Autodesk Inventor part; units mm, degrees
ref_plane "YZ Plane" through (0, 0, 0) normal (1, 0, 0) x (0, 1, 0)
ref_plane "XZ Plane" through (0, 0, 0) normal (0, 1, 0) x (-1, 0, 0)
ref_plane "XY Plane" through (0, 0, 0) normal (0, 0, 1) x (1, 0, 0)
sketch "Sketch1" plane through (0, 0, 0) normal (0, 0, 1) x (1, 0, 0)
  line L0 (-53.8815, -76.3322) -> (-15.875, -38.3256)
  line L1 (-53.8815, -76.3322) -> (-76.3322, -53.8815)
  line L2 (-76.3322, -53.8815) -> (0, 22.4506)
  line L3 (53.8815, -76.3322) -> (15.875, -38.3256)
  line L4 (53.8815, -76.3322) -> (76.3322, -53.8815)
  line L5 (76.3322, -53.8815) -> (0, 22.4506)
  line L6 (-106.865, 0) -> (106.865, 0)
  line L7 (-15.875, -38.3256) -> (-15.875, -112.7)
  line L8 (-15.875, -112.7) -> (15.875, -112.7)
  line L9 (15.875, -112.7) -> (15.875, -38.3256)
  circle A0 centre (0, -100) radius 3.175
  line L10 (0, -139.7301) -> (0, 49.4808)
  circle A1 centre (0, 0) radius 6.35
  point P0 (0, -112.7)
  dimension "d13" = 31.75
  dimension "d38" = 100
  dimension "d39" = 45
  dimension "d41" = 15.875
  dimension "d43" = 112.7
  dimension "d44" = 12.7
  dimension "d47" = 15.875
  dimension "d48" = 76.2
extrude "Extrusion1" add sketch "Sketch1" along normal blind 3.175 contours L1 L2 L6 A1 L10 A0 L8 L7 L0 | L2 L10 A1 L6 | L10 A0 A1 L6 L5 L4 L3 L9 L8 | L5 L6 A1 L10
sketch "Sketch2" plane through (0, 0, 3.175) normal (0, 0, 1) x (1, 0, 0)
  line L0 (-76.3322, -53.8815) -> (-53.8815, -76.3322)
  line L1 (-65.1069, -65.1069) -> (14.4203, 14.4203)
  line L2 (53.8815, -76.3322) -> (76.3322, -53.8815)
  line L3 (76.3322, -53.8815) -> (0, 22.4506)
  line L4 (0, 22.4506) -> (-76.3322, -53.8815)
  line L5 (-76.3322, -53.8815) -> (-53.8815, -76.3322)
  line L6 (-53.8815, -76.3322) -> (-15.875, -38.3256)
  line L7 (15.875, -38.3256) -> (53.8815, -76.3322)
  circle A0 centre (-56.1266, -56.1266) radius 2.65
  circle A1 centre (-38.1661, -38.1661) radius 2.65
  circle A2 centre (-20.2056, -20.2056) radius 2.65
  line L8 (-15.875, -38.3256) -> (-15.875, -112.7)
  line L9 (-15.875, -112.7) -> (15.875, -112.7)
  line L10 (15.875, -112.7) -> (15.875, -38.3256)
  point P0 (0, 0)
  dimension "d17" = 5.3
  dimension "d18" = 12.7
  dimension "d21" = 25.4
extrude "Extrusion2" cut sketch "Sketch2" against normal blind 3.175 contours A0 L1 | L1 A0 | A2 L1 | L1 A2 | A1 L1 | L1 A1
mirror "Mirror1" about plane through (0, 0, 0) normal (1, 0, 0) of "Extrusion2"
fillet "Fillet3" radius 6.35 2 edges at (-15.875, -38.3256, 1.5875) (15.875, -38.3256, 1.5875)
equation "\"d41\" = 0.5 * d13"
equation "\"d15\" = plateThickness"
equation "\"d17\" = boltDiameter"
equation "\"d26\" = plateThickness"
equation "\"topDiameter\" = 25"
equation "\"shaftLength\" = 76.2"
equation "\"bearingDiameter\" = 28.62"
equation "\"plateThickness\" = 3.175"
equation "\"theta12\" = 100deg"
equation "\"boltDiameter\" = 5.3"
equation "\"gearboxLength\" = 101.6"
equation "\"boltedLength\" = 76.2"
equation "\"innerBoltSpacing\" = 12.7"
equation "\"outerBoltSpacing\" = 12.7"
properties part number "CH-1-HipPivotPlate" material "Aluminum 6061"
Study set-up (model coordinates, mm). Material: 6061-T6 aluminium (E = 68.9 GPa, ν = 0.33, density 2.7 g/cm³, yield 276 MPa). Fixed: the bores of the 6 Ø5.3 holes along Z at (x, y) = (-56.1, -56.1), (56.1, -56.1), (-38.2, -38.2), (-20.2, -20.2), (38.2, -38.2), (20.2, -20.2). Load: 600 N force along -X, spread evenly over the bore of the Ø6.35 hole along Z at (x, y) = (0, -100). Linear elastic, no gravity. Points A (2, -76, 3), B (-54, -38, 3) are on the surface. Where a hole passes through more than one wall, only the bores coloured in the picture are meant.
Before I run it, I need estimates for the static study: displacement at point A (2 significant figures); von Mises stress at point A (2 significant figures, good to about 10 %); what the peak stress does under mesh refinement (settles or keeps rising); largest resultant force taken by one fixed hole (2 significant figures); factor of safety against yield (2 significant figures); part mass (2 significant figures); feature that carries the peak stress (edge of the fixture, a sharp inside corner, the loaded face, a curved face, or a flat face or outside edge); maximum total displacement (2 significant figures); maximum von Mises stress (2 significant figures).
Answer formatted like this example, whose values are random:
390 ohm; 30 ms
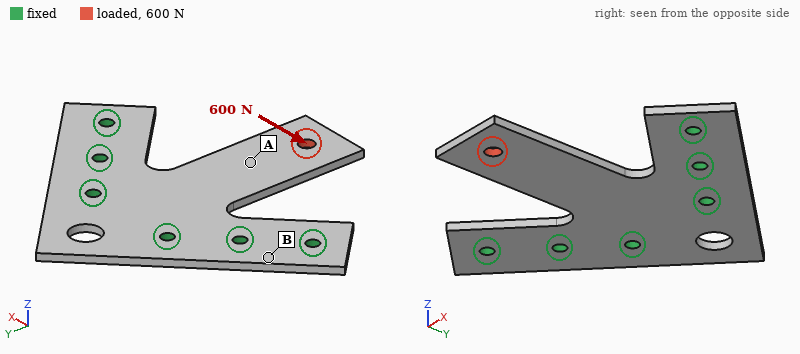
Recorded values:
0.040 mm; 16 MPa; settles; 530 N; 3.0; 71 g; a curved face; 0.12 mm; 92 MPa
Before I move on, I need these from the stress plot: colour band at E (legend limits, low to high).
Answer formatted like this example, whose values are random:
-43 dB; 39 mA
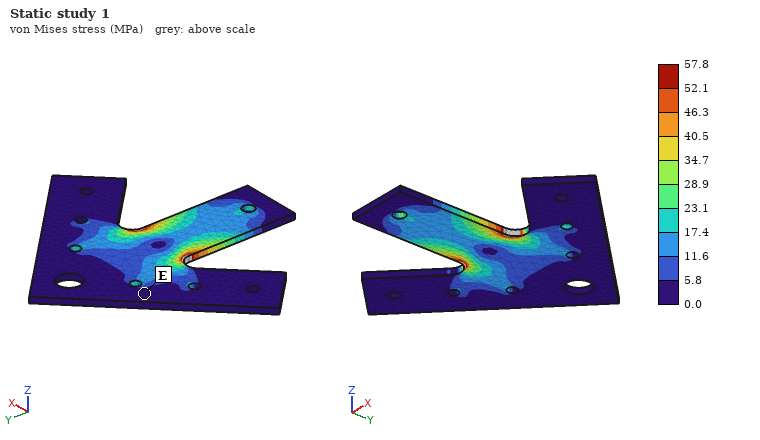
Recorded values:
0.0 to 5.8 MPa
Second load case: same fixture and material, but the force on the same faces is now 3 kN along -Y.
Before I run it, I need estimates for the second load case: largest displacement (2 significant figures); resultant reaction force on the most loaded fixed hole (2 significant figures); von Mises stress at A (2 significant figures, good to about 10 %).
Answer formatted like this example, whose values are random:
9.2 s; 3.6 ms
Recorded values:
40 µm; 1.3 kN; 32 MPa
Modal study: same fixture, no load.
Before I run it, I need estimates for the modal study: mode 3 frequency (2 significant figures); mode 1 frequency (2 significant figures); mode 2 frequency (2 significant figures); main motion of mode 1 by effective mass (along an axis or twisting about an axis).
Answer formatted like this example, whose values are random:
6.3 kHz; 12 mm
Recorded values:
2300 Hz; 430 Hz; 2200 Hz; along Z
